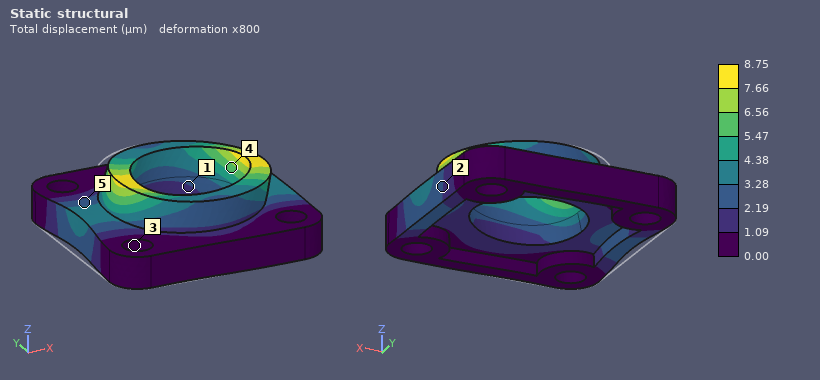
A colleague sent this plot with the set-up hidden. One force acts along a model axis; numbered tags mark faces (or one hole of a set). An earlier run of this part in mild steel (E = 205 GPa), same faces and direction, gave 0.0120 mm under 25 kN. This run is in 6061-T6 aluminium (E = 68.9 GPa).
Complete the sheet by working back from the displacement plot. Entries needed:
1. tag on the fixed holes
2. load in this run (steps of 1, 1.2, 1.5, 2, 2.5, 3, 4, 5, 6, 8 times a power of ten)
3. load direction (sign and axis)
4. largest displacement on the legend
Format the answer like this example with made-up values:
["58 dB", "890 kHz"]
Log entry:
["3", "6 kN", "+X", "8.75 µm"]
